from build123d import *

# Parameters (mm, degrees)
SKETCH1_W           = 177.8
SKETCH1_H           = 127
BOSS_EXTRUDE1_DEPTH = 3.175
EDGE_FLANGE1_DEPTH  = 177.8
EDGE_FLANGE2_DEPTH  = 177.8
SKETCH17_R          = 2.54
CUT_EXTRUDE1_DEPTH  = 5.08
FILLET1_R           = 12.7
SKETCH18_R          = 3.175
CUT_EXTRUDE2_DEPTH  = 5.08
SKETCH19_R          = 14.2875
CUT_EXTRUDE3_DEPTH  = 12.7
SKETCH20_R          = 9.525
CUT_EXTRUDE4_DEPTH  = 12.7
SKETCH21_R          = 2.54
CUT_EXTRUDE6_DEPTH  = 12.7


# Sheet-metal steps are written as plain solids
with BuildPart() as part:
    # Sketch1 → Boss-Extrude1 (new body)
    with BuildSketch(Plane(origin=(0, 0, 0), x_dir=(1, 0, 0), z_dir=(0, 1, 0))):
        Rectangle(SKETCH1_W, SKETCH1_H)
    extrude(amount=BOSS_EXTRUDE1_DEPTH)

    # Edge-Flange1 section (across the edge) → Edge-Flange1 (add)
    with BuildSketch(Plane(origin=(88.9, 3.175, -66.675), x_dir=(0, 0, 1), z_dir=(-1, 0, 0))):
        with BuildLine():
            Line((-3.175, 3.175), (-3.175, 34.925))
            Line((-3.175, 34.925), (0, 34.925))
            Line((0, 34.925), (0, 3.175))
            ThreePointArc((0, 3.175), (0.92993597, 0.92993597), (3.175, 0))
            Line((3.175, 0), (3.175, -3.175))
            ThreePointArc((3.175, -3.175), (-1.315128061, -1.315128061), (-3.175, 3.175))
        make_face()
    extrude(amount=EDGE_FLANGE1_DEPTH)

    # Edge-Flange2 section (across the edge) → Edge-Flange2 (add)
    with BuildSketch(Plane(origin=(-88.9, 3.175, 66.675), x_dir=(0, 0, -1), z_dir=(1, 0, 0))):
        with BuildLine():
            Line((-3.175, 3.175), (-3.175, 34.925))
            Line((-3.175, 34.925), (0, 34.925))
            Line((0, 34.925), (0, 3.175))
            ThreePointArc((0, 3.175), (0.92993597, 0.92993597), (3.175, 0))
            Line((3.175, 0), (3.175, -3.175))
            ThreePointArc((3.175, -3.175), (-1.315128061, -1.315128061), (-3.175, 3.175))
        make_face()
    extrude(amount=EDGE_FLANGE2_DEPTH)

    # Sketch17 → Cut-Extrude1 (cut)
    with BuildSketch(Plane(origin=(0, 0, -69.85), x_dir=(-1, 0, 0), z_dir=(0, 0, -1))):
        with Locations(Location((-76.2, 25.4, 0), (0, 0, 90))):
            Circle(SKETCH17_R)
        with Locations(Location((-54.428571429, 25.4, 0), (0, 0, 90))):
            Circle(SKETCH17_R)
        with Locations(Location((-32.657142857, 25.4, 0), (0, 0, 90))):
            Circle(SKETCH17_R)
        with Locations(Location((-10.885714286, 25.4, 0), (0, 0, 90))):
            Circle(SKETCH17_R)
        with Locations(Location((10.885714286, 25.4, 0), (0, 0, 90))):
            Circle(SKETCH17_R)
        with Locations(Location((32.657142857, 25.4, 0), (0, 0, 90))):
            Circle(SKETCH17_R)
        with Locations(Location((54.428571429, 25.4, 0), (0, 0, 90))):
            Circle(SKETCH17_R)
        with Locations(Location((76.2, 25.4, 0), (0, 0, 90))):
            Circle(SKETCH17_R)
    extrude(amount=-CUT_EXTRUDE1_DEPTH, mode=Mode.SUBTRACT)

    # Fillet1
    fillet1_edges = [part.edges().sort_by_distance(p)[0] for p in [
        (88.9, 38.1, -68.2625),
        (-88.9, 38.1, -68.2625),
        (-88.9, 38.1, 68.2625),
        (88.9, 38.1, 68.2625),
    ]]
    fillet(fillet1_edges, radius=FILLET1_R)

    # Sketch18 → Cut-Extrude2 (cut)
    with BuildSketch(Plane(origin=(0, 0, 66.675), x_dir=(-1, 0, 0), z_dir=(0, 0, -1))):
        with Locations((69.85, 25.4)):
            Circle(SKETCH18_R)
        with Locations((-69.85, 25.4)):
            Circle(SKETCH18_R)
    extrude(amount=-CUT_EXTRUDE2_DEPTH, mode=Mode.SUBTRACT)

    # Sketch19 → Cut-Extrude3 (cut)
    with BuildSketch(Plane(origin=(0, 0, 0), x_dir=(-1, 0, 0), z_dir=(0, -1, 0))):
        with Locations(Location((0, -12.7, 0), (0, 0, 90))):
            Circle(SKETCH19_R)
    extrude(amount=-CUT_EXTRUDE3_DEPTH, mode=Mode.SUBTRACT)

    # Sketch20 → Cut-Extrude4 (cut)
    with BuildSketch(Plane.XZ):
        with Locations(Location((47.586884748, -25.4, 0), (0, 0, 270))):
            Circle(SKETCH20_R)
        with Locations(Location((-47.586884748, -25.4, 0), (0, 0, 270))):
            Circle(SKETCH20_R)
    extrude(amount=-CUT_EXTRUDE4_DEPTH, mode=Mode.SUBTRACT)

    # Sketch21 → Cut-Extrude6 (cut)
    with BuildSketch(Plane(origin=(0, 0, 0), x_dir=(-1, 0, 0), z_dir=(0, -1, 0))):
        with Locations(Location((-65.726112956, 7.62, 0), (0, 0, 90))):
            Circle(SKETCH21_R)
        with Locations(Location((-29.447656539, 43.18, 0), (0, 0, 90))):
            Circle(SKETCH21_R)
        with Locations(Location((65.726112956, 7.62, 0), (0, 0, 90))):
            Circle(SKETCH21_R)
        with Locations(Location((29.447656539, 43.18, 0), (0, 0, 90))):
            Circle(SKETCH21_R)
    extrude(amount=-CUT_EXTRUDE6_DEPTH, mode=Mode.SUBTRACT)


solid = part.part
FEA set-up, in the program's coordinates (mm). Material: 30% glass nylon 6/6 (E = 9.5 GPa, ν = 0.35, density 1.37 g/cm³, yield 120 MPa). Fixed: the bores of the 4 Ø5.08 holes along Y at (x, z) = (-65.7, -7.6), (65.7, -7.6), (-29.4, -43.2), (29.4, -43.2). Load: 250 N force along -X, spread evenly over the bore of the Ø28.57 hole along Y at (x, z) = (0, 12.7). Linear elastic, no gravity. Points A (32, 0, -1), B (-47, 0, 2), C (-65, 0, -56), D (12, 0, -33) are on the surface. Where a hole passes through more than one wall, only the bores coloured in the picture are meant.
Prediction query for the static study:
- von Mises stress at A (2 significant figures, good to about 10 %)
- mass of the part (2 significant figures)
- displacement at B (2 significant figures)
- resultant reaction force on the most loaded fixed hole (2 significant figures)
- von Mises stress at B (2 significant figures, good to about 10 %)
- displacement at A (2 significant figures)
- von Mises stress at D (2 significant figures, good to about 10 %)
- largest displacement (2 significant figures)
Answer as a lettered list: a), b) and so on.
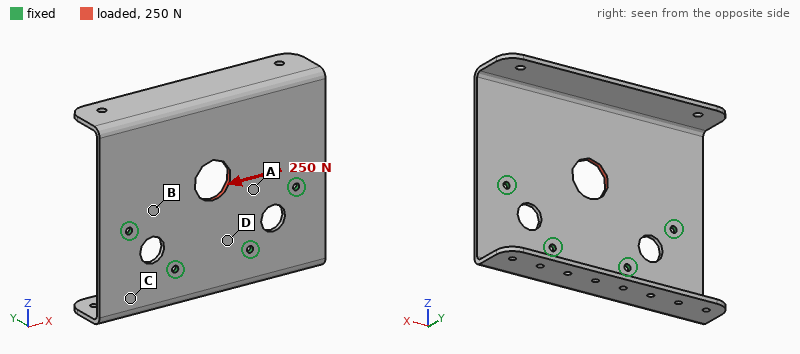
a) 0.85 MPa
b) 150 g
c) 3.2 µm
d) 100 N
e) 1.0 MPa
f) 3.8 µm
g) 0.49 MPa
h) 9.2 µm
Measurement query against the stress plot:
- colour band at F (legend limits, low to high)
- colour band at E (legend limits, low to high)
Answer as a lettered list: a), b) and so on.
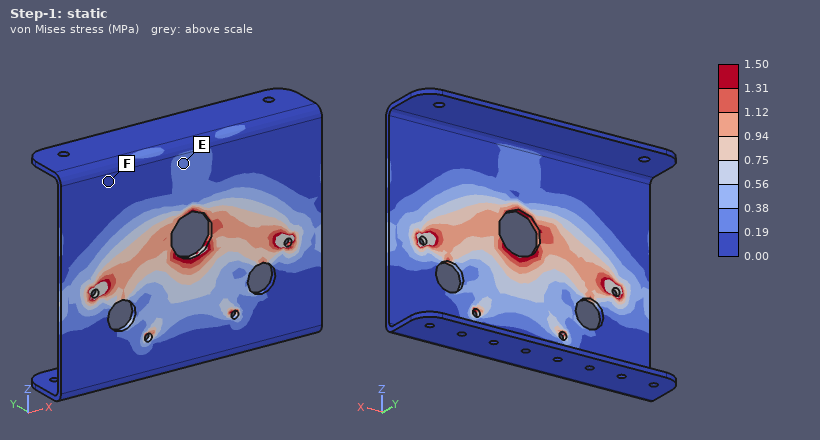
a) 0.00 to 0.19 MPa
b) 0.19 to 0.38 MPa
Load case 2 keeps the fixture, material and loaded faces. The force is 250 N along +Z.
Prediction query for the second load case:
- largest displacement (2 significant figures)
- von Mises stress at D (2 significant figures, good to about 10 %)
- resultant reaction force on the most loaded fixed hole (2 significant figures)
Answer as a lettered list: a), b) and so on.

a) 7.8 µm
b) 0.53 MPa
c) 80 N
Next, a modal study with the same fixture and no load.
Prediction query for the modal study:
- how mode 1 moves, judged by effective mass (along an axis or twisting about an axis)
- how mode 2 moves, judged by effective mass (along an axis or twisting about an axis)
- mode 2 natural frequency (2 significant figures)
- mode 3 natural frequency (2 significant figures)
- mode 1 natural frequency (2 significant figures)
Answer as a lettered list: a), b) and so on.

a) along Y
b) twisting about Z
c) 210 Hz
d) 420 Hz
e) 120 Hz
